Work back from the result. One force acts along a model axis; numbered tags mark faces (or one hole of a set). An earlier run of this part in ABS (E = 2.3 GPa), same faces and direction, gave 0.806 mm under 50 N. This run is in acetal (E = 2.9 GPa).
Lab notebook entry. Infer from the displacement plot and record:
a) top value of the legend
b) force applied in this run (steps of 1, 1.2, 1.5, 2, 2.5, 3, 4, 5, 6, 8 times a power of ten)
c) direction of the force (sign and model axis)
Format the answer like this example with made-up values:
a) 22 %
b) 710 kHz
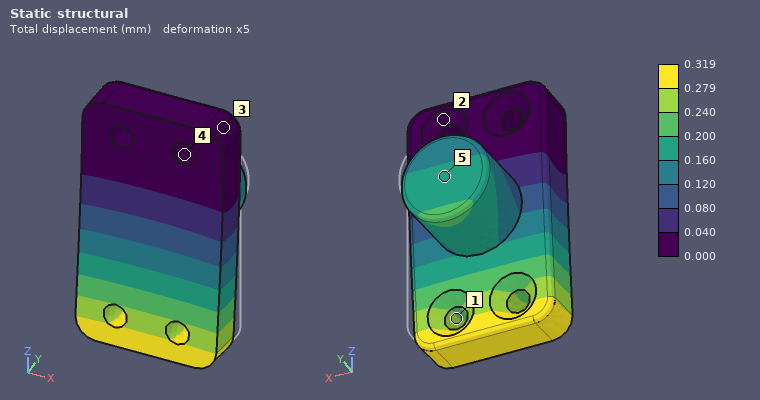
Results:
a) 0.319 mm
b) 25 N
c) -Y
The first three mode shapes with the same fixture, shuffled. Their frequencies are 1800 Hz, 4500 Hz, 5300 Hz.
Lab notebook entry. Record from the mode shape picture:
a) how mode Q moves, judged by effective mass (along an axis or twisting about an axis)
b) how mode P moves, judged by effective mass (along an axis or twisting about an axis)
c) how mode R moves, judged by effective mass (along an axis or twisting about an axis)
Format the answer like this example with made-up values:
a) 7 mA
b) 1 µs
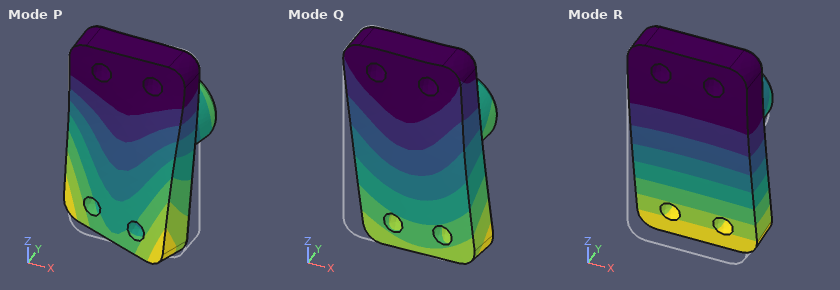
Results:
a) along X
b) twisting about Z
c) along Y
